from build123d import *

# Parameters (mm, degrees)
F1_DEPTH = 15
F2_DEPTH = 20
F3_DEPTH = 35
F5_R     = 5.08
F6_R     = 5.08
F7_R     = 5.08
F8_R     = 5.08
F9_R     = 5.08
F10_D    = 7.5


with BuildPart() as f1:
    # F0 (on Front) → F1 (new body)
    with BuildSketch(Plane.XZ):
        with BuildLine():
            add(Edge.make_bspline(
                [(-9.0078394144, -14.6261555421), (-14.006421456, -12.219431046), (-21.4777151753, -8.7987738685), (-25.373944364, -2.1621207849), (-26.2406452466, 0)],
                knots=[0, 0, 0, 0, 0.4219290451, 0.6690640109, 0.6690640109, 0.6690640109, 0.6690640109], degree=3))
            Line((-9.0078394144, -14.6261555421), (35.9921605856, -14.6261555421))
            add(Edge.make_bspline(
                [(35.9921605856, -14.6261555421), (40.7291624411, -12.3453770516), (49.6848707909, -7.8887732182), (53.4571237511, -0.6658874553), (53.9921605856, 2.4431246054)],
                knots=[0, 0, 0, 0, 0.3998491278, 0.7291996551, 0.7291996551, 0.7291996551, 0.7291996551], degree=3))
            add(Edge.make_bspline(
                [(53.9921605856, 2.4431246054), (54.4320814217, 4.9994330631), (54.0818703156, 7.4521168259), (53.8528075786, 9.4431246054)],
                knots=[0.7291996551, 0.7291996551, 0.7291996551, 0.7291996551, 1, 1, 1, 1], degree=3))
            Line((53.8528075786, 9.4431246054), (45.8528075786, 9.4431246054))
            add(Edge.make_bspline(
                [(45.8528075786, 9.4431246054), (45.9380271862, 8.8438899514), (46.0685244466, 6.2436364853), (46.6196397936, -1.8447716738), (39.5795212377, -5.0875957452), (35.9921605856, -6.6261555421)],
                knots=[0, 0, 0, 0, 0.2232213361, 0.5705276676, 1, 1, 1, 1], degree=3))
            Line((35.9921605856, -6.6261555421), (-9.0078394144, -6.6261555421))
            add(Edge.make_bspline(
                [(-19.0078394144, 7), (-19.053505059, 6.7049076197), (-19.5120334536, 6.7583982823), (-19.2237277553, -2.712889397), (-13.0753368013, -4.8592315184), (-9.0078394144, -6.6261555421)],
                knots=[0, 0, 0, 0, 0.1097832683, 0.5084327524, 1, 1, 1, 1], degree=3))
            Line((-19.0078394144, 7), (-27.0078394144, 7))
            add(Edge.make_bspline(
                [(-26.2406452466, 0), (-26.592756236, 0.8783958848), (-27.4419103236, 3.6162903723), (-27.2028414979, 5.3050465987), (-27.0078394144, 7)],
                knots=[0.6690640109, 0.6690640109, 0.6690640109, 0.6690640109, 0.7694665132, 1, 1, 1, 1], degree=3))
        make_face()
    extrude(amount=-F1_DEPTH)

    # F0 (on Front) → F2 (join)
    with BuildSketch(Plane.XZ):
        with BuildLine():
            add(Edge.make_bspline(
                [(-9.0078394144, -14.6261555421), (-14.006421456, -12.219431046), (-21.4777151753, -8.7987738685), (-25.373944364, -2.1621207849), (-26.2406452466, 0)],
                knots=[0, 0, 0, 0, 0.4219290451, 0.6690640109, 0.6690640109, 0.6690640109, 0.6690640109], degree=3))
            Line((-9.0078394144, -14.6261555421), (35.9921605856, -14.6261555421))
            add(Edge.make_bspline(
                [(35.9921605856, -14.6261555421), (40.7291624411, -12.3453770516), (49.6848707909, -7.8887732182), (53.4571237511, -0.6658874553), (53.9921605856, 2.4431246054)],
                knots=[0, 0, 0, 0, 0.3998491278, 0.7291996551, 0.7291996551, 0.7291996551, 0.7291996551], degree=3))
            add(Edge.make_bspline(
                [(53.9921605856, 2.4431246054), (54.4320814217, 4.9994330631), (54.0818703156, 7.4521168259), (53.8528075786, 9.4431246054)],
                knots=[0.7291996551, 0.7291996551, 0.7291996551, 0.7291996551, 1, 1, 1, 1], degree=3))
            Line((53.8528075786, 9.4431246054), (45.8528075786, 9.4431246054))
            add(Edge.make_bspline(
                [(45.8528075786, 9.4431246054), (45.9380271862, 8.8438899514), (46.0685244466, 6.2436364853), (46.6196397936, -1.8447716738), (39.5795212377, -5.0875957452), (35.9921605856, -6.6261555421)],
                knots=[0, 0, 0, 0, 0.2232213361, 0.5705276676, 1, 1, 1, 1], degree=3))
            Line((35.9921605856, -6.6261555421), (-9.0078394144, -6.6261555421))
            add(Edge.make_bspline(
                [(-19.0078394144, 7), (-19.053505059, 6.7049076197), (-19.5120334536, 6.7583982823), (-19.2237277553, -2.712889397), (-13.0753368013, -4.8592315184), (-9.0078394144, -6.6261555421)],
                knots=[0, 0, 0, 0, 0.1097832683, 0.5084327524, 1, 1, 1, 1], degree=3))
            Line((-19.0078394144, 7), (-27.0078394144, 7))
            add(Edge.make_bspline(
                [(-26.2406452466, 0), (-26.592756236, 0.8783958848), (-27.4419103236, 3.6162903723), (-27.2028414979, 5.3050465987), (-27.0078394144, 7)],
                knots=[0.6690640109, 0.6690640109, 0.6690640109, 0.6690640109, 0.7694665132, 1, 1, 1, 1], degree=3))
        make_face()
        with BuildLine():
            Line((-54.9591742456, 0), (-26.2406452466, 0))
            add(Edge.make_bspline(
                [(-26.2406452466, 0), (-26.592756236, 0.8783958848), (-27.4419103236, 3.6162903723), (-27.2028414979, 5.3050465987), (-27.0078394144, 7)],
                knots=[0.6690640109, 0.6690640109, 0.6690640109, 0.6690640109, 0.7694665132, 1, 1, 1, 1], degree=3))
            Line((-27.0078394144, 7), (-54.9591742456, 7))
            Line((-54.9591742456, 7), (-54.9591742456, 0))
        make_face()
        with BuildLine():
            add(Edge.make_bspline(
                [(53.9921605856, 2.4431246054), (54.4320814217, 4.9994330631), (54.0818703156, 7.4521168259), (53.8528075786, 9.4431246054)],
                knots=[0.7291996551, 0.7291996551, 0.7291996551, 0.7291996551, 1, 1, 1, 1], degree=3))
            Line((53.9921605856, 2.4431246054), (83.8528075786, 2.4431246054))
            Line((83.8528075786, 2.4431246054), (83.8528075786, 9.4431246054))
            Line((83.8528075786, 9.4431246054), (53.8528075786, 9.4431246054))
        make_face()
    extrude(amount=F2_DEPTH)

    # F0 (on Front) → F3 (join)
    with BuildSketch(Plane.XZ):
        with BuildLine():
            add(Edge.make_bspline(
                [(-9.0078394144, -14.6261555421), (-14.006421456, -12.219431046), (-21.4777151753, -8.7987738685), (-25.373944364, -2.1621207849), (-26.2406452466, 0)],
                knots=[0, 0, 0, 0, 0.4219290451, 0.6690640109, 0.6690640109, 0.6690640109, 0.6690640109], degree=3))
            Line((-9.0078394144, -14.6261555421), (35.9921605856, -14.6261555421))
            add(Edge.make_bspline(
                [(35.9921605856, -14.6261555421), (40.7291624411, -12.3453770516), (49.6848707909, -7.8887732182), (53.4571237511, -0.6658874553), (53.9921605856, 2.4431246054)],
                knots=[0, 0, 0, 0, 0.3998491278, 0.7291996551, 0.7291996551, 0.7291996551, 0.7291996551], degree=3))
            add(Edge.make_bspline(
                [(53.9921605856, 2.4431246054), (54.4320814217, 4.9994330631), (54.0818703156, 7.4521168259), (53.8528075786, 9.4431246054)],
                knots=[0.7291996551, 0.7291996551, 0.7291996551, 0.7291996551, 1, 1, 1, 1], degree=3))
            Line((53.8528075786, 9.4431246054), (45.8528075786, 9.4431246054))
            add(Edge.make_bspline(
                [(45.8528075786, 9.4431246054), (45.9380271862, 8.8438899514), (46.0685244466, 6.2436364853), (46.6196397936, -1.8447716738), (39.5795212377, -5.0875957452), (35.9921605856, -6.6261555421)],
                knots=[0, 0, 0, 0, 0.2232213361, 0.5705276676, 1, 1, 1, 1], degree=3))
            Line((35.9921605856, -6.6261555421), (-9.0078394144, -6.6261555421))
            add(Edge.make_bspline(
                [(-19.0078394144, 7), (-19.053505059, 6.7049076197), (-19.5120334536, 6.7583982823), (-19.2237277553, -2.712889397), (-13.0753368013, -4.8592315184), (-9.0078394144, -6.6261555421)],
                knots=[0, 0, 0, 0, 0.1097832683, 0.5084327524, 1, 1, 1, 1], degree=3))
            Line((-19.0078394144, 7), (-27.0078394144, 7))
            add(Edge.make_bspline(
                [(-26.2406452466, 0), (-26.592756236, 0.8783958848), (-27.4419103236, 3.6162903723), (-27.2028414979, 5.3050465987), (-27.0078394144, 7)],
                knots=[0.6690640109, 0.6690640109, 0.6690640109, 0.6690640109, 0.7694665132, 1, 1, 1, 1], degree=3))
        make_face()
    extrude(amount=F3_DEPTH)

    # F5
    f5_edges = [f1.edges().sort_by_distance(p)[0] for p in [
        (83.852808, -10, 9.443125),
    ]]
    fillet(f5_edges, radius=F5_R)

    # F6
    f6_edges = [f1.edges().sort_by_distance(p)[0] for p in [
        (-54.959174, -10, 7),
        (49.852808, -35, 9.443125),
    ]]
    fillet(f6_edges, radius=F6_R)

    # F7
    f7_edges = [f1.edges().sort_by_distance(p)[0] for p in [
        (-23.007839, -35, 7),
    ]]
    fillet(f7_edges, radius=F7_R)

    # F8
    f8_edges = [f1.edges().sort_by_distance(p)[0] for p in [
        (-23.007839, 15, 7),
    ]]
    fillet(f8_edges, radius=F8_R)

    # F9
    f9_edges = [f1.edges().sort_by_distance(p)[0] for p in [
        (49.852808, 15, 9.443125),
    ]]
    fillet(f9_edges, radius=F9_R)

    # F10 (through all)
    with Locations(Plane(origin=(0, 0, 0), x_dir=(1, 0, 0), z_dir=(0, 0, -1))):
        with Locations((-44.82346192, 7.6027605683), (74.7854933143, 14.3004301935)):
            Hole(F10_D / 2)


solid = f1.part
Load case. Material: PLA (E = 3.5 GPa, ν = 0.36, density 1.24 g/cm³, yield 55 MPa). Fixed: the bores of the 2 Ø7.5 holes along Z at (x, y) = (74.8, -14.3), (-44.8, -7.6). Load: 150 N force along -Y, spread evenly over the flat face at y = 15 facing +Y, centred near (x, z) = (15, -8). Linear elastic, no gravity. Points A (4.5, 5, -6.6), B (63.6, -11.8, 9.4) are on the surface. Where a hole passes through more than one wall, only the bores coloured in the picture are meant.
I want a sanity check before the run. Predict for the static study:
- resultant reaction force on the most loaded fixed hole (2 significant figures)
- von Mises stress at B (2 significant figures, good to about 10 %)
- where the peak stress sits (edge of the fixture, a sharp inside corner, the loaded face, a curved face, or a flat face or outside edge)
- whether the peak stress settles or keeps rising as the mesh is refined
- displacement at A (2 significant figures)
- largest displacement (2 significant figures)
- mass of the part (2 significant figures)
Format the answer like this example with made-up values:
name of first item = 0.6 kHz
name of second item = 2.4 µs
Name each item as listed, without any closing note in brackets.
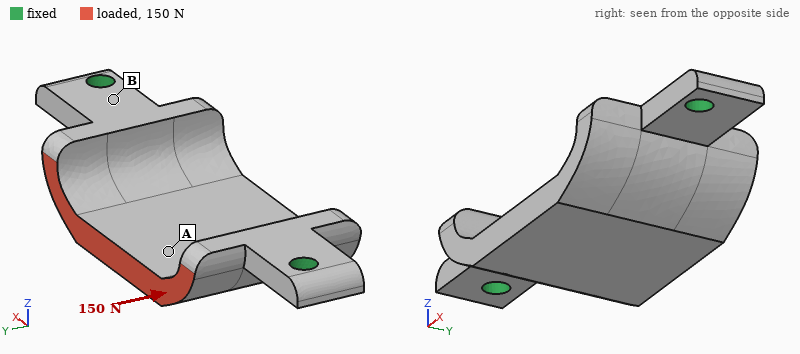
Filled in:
resultant reaction force on the most loaded fixed hole = 78 N
von Mises stress at B = 3.6 MPa
where the peak stress sits = edge of the fixture
whether the peak stress settles or keeps rising as the mesh is refined = keeps rising
displacement at A = 0.19 mm
largest displacement = 0.31 mm
mass of the part = 54 g
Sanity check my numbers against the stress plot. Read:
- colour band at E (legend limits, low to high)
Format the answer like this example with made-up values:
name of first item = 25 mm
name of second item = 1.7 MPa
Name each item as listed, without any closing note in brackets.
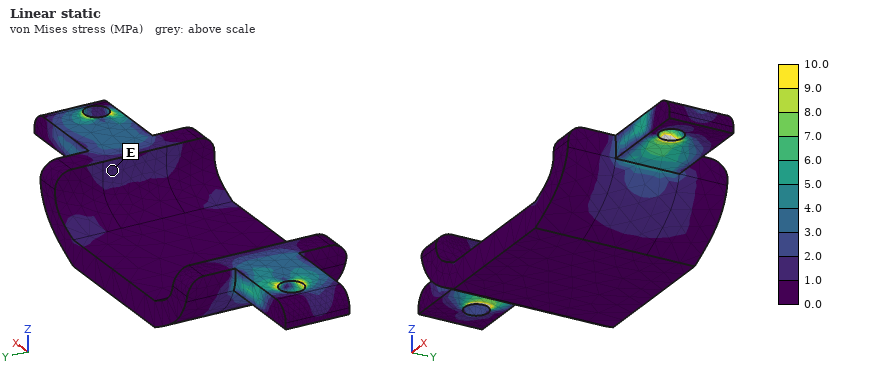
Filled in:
colour band at E = 1.0 to 2.0 MPa
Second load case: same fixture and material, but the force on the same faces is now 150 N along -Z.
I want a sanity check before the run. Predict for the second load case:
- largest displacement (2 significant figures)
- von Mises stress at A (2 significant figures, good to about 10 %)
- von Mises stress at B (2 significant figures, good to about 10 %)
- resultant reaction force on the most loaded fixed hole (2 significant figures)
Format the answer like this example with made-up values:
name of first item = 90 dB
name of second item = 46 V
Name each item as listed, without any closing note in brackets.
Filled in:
largest displacement = 0.59 mm
von Mises stress at A = 1.4 MPa
von Mises stress at B = 9.6 MPa
resultant reaction force on the most loaded fixed hole = 140 N
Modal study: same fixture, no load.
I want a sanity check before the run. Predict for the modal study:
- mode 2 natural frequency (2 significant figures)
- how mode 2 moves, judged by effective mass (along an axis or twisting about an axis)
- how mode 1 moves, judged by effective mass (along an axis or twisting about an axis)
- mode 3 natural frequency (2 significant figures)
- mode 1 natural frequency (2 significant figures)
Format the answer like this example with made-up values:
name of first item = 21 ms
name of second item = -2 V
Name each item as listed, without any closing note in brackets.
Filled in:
mode 2 natural frequency = 1200 Hz
how mode 2 moves, judged by effective mass = along Z
how mode 1 moves, judged by effective mass = along Y
mode 3 natural frequency = 1600 Hz
mode 1 natural frequency = 580 Hz
